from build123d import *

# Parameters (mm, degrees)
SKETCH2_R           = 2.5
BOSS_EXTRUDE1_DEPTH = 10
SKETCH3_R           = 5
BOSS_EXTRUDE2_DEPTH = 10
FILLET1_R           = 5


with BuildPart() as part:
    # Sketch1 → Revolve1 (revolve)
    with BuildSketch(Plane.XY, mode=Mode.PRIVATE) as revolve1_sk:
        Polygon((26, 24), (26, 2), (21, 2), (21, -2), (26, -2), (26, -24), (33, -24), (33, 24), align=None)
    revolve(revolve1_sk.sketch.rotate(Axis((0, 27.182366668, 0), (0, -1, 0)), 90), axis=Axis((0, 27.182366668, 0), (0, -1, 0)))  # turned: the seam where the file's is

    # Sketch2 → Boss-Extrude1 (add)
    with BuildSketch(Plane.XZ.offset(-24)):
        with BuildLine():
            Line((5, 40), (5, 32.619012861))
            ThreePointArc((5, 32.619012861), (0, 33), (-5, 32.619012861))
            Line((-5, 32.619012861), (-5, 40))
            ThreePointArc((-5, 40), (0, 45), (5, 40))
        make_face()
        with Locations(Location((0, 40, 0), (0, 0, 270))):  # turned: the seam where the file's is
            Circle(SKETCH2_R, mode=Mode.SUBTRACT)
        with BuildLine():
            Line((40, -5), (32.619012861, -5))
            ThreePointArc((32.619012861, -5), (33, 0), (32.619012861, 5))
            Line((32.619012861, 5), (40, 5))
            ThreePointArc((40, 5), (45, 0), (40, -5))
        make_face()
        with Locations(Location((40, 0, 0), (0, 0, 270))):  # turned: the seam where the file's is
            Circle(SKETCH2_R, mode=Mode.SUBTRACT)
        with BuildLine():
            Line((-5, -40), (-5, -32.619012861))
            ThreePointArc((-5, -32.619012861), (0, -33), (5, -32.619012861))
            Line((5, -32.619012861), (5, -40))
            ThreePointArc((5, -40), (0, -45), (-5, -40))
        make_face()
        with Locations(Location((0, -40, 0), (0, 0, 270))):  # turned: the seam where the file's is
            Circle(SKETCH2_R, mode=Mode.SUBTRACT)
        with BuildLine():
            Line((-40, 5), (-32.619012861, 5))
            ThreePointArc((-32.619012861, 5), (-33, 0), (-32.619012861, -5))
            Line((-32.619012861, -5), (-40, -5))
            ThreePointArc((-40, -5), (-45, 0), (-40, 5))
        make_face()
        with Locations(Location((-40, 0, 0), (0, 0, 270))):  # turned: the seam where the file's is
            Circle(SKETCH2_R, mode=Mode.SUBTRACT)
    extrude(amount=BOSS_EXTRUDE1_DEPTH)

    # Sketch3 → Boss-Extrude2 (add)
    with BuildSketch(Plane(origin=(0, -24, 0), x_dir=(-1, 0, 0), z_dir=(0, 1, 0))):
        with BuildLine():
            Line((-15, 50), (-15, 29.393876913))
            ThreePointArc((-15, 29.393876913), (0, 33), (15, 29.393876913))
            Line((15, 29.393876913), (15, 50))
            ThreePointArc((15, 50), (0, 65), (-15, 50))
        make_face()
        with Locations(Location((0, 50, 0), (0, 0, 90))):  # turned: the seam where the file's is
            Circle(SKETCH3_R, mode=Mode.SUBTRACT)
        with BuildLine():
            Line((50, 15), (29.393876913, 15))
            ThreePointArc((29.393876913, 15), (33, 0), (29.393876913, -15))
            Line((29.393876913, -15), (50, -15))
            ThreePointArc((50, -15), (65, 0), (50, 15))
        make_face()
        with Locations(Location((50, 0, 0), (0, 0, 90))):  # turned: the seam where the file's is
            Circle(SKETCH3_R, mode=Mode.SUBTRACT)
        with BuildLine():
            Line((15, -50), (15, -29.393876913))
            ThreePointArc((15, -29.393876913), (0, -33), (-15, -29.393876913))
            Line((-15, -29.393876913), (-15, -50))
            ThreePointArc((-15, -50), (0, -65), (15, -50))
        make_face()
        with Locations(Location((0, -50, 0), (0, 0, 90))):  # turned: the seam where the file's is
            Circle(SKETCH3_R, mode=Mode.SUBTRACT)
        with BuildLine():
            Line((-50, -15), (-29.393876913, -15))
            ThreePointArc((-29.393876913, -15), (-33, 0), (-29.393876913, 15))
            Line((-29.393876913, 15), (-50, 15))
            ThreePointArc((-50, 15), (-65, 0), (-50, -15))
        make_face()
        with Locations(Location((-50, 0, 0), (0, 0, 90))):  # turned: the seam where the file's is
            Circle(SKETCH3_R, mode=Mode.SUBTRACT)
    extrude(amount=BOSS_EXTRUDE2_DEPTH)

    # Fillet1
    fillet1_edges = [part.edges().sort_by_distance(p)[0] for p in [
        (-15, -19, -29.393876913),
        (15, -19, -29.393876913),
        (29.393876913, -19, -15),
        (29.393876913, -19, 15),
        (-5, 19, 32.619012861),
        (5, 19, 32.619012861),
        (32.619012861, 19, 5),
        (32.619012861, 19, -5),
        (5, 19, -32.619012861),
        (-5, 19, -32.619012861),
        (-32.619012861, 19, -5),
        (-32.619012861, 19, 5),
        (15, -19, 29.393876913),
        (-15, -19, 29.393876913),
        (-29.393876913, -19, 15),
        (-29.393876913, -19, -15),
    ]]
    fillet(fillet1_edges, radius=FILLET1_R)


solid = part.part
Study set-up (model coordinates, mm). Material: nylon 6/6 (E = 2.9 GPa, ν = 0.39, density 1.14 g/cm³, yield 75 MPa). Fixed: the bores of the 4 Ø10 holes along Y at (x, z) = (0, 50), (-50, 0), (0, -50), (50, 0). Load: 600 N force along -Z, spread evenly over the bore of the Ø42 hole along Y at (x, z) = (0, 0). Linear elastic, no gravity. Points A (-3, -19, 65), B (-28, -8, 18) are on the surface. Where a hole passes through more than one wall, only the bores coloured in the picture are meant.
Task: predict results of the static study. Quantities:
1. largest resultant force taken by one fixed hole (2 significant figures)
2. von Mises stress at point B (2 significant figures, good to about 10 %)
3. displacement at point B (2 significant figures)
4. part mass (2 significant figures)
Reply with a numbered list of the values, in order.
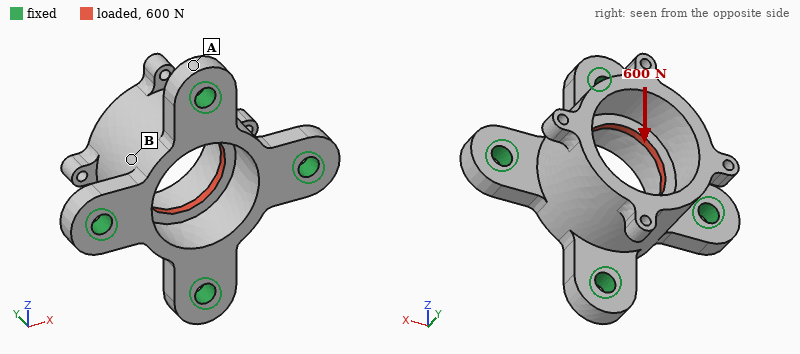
1. 250 N
2. 0.74 MPa
3. 27 µm
4. 120 g
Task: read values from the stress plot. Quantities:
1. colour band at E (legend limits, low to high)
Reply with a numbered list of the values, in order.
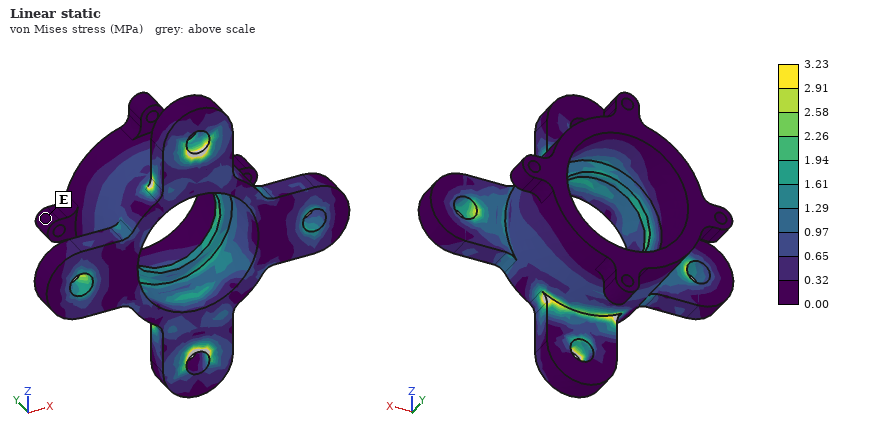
1. 0.00 to 0.32 MPa
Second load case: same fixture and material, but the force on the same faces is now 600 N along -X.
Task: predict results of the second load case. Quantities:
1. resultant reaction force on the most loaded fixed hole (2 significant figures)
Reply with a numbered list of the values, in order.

1. 250 N
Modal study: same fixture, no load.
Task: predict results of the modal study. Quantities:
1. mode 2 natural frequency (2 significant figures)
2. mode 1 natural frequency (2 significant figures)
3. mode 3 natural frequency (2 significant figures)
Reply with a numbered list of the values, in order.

1. 1900 Hz
2. 1900 Hz
3. 2300 Hz
